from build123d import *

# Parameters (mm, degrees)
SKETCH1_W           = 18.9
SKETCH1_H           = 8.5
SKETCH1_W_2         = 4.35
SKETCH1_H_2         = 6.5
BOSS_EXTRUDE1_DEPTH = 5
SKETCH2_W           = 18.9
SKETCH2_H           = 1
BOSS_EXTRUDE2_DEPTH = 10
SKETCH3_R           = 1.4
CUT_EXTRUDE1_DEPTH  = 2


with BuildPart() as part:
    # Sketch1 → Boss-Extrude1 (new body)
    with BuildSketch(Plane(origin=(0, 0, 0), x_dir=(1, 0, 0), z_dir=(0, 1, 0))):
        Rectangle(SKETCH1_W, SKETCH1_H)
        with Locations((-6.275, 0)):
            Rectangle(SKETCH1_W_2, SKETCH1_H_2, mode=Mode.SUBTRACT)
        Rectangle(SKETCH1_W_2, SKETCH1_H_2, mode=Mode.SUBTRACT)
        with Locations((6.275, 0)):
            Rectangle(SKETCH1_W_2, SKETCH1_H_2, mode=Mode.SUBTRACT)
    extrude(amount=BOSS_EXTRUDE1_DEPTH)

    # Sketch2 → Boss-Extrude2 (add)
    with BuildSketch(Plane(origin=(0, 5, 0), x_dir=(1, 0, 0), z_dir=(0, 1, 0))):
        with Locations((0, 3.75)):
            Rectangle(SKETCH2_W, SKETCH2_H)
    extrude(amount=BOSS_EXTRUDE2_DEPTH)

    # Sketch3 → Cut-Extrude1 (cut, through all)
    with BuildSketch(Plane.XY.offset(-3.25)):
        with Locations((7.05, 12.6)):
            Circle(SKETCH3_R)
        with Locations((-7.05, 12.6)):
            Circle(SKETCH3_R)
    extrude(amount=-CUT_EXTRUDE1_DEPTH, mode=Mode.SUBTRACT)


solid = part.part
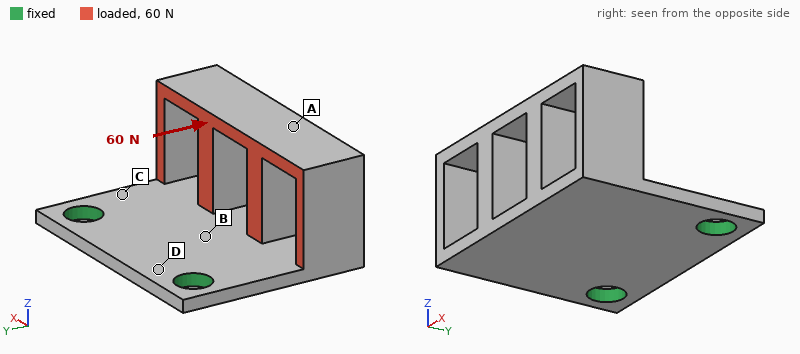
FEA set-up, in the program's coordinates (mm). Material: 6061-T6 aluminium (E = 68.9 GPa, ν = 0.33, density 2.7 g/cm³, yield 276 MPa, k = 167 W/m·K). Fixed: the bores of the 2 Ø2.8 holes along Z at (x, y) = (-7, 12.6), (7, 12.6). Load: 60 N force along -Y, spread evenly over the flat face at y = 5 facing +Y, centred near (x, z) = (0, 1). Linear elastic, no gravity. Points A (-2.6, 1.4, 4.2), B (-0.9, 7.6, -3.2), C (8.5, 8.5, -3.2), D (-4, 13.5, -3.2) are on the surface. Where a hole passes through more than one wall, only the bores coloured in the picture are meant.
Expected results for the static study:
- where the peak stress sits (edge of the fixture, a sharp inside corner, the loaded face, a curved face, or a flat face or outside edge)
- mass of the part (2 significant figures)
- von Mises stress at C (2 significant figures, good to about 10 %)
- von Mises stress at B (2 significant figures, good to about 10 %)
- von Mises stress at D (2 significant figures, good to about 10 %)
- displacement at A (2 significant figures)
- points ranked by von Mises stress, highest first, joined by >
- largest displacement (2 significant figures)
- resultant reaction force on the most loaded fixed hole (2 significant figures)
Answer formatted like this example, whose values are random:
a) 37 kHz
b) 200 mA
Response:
a) a flat face or outside edge
b) 1.5 g
c) 110 MPa
d) 82 MPa
e) 29 MPa
f) 0.22 mm
g) C > B > D > A
h) 0.24 mm
i) 31 N
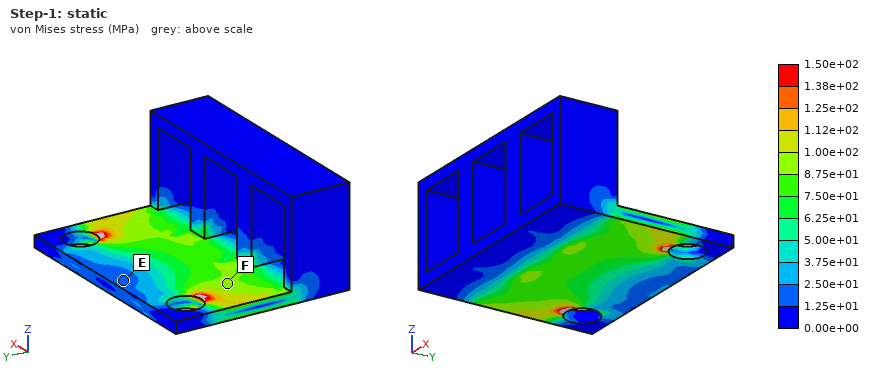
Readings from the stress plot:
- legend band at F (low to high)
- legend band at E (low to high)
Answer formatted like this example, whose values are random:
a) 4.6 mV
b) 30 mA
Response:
a) 8.75e+01 to 1.00e+02 MPa
b) 1.25e+01 to 2.50e+01 MPa
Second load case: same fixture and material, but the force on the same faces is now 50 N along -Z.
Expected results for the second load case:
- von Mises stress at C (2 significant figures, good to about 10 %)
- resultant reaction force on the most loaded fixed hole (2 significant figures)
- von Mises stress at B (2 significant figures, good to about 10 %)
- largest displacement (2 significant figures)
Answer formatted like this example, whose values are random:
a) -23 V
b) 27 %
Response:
a) 67 MPa
b) 25 N
c) 33 MPa
d) 0.14 mm
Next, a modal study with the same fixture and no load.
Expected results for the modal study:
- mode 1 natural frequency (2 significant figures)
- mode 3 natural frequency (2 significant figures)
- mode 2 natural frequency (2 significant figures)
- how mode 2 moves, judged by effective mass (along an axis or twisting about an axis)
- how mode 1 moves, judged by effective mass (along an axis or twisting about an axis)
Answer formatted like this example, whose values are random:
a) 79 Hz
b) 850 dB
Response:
a) 2400 Hz
b) 11 kHz
c) 6000 Hz
d) along X
e) along Z
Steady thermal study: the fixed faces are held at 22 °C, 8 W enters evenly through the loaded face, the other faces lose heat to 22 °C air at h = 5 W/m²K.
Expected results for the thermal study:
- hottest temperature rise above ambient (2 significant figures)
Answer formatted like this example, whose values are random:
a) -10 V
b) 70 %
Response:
a) 33 K
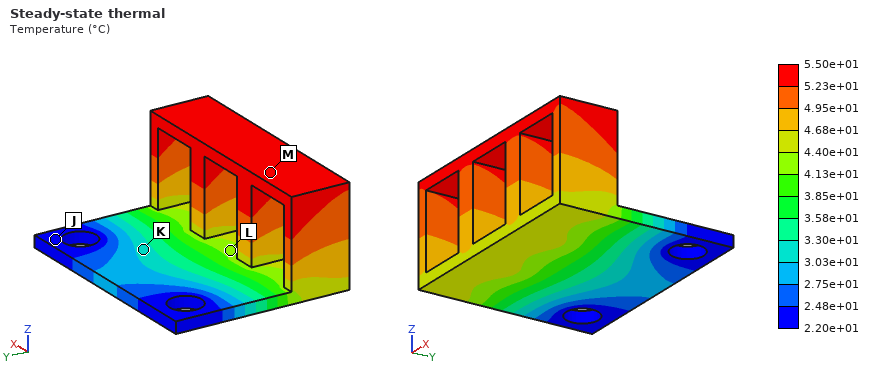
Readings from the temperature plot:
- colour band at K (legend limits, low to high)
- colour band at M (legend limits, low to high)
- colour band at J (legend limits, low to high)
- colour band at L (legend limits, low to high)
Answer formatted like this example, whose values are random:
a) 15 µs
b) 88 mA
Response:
a) 3.03e+01 to 3.30e+01 °C
b) 5.23e+01 to 5.50e+01 °C
c) 2.20e+01 to 2.48e+01 °C
d) 4.13e+01 to 4.40e+01 °C
